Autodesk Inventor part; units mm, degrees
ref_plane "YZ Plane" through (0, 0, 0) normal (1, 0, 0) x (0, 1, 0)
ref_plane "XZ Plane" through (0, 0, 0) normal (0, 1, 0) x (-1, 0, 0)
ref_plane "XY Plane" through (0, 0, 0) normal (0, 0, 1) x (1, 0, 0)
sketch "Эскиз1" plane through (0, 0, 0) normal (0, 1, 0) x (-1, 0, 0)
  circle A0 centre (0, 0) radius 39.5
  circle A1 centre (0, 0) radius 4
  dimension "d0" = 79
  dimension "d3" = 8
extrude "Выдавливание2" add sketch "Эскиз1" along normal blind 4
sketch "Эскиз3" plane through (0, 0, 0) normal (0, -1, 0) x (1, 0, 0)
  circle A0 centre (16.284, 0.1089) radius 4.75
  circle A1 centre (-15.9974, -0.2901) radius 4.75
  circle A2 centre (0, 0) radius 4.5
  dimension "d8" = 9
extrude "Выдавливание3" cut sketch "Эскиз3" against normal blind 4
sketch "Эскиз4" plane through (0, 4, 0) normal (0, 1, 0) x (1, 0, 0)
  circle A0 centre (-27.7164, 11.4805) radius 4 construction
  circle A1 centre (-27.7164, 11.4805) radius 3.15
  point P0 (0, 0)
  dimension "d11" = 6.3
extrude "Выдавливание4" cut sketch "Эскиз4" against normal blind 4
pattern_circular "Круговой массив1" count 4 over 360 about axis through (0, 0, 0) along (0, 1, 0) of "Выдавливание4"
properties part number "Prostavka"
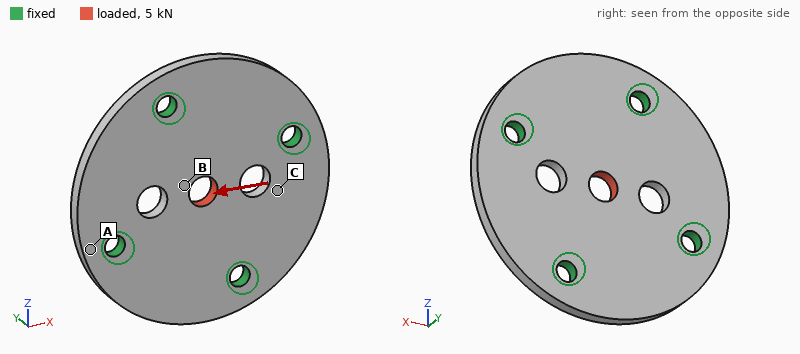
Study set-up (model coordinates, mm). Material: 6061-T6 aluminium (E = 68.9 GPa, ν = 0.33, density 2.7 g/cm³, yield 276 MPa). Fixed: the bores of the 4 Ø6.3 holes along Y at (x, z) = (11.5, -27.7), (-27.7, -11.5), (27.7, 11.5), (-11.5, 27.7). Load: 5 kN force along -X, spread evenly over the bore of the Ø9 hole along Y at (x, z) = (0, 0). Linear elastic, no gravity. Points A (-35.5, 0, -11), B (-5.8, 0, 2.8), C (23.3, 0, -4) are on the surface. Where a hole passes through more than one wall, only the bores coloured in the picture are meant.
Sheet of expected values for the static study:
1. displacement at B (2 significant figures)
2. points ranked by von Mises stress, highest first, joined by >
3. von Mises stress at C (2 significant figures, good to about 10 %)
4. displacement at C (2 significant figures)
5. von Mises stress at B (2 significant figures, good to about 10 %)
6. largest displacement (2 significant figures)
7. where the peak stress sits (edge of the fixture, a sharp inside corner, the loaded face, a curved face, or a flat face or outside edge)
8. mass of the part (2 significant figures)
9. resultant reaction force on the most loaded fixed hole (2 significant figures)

13 µm
B > C > A
16 MPa
4.6 µm
42 MPa
15 µm
a curved face
49 g
1.5 kN
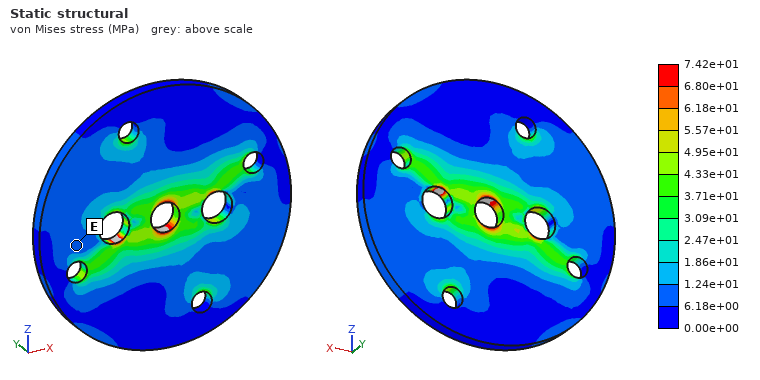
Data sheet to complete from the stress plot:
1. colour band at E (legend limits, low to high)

6.18e+00 to 1.24e+01 MPa
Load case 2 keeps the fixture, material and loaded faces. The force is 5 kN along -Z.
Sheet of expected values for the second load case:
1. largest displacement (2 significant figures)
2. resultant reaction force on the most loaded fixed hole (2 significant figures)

12 µm
1.6 kN
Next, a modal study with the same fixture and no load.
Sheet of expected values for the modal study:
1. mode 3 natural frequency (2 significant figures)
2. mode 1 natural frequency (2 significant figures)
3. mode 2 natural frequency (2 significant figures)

8800 Hz
8500 Hz
8700 Hz
